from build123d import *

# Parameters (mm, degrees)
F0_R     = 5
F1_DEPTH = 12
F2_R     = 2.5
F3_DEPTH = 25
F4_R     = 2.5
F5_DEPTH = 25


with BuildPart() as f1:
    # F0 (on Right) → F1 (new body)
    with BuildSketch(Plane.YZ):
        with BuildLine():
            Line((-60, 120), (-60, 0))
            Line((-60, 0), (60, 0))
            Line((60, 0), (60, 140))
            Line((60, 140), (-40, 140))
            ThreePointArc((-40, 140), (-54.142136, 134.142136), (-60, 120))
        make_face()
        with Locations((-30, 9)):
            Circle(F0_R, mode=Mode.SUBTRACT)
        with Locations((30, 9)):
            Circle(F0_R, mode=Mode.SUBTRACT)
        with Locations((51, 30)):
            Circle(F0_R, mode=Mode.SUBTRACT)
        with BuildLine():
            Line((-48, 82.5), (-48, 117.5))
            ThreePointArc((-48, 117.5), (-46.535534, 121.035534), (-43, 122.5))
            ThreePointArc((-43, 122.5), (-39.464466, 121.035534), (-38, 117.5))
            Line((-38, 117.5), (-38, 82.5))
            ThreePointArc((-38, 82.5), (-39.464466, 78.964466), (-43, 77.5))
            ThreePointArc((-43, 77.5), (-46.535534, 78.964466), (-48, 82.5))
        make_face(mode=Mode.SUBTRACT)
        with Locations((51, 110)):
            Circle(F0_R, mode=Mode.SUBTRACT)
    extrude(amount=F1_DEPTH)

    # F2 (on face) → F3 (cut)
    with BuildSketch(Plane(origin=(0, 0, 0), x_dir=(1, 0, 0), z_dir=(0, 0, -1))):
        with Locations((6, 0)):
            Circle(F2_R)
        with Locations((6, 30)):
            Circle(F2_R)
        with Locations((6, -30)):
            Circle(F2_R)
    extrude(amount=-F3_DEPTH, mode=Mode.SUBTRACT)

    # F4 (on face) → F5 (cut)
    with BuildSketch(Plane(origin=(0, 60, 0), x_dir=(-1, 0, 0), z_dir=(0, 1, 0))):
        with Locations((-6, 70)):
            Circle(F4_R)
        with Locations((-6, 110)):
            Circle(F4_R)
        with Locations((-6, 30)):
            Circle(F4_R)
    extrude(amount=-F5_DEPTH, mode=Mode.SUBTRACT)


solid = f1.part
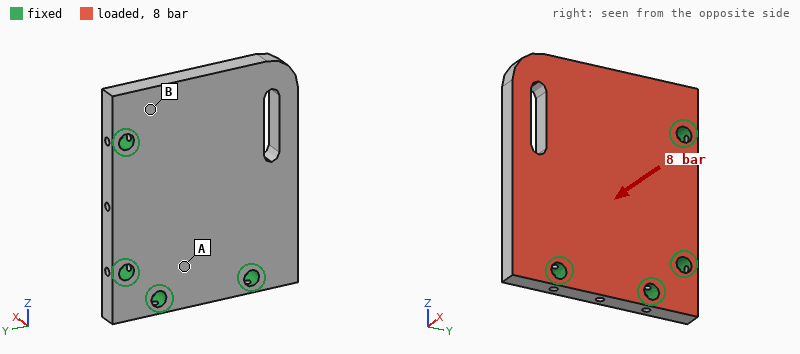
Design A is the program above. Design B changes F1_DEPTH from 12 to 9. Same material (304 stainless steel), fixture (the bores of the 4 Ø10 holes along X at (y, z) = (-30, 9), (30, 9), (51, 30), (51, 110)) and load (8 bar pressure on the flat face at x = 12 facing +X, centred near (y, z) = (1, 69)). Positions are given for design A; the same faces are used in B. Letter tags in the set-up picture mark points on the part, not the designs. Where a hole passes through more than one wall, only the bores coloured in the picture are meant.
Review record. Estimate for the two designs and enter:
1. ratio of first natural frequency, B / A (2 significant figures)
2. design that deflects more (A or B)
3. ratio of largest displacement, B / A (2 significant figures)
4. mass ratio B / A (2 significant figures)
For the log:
0.77
B
2.3
0.75
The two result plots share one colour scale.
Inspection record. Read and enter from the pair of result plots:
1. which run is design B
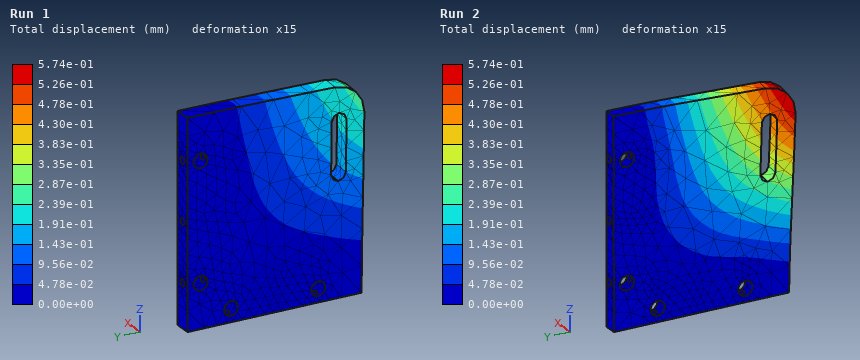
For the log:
Run 2
